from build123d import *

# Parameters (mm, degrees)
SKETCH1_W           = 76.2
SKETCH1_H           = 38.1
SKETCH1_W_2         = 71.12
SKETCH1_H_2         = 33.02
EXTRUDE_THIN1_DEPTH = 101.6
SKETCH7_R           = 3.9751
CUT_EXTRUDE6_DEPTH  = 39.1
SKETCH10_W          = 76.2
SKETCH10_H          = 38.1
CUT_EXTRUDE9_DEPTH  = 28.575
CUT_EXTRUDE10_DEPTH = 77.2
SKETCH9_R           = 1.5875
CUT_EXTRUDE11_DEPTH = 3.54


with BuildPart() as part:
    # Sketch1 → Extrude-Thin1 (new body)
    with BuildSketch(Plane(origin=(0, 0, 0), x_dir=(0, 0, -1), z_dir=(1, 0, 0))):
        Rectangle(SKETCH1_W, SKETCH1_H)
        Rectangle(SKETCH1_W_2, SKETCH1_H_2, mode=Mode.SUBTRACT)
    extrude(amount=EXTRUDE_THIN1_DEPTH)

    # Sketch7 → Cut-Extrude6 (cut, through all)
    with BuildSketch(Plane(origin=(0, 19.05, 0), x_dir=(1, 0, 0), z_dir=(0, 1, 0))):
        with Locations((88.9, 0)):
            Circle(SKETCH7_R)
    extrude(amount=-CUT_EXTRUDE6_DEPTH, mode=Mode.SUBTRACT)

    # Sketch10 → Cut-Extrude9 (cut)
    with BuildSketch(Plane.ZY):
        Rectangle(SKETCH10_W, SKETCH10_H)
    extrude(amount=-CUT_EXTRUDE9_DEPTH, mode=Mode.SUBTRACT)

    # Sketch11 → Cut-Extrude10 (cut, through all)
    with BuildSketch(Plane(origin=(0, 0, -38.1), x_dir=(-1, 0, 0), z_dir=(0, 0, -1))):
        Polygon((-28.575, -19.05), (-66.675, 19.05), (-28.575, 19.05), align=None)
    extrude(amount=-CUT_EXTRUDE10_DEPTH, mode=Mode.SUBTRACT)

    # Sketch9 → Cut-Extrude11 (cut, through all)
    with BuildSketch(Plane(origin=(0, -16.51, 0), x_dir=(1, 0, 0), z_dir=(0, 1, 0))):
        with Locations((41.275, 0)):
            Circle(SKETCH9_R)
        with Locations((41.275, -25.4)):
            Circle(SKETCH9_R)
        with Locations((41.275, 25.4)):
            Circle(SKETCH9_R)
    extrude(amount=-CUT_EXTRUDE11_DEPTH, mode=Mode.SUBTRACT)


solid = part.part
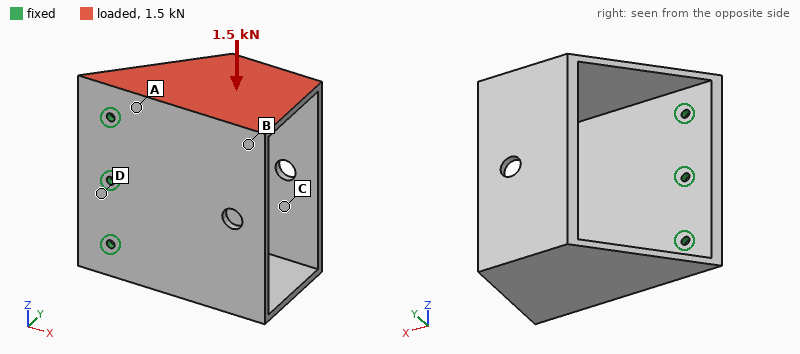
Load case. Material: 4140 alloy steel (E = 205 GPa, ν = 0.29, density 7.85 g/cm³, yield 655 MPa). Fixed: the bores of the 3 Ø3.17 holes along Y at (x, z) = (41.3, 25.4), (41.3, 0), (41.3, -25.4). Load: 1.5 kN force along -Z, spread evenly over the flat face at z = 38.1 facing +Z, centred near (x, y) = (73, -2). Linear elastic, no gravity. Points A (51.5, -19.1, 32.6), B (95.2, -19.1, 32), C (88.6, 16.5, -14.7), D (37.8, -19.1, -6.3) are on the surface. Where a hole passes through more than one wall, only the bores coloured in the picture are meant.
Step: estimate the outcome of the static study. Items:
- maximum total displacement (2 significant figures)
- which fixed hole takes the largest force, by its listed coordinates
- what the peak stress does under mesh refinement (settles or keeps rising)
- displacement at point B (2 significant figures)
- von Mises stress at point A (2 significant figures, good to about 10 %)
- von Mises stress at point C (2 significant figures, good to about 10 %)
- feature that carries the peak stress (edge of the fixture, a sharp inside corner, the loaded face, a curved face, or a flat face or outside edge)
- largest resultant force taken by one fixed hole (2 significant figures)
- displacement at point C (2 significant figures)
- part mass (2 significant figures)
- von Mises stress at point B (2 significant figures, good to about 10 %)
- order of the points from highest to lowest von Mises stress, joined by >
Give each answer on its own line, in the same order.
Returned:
0.45 mm
(41.3, 25.4)
keeps rising
0.16 mm
130 MPa
50 MPa
edge of the fixture
1.2 kN
0.34 mm
230 g
71 MPa
A > B > C > D
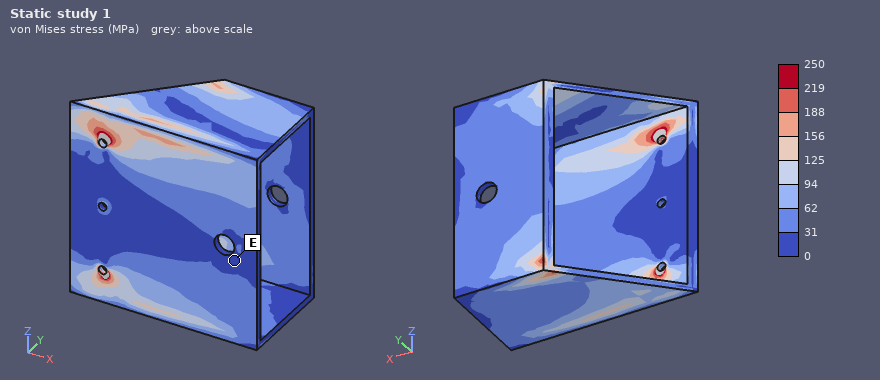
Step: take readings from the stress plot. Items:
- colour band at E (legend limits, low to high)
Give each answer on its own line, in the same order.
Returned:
0 to 31 MPa
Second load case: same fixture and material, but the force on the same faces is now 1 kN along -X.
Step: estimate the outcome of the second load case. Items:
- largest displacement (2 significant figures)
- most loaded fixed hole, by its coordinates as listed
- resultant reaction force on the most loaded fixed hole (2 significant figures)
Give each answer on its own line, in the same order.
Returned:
0.54 mm
(41.3, 25.4)
1.2 kN
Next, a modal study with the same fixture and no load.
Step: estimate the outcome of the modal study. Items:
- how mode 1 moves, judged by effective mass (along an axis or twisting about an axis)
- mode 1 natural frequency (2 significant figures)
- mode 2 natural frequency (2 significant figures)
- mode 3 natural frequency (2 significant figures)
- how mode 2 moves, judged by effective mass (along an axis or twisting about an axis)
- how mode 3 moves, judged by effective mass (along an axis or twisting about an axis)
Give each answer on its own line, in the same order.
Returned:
along Y
430 Hz
660 Hz
1200 Hz
along Z
along Z
